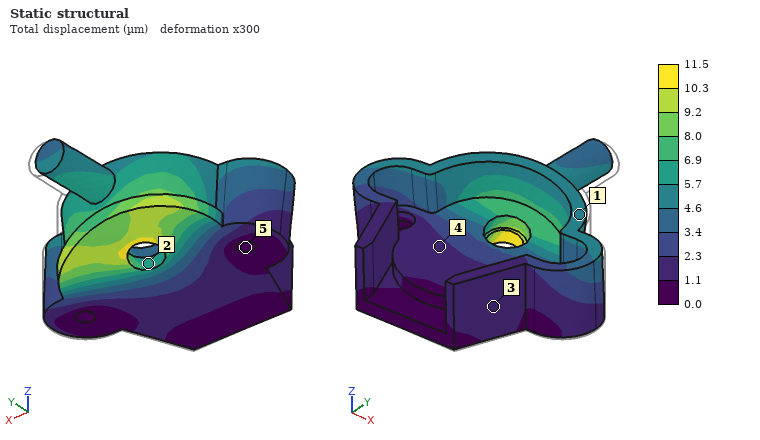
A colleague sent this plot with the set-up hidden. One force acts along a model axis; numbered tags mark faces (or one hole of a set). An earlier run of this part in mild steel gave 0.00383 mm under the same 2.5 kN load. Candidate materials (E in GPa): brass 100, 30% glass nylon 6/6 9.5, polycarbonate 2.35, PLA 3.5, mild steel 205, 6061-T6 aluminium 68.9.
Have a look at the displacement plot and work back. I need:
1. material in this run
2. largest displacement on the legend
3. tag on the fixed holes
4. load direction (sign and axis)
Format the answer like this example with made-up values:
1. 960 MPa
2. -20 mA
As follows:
1. 6061-T6 aluminium
2. 11.5 µm
3. 5
4. -X
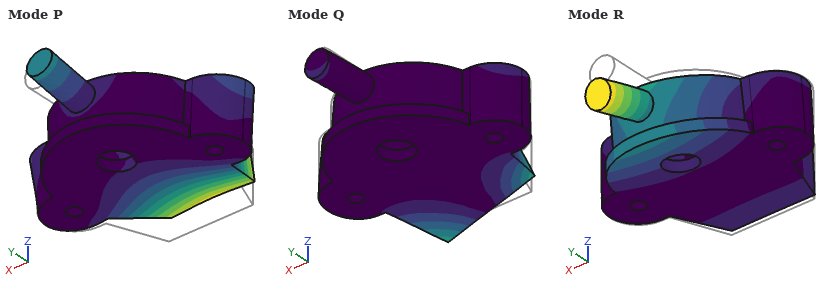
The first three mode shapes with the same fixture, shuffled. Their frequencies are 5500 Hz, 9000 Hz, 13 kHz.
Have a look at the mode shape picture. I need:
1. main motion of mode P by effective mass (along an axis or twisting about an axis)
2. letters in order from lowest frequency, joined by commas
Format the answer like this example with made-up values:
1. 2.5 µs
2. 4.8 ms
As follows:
1. along Z
2. R, P, Q
